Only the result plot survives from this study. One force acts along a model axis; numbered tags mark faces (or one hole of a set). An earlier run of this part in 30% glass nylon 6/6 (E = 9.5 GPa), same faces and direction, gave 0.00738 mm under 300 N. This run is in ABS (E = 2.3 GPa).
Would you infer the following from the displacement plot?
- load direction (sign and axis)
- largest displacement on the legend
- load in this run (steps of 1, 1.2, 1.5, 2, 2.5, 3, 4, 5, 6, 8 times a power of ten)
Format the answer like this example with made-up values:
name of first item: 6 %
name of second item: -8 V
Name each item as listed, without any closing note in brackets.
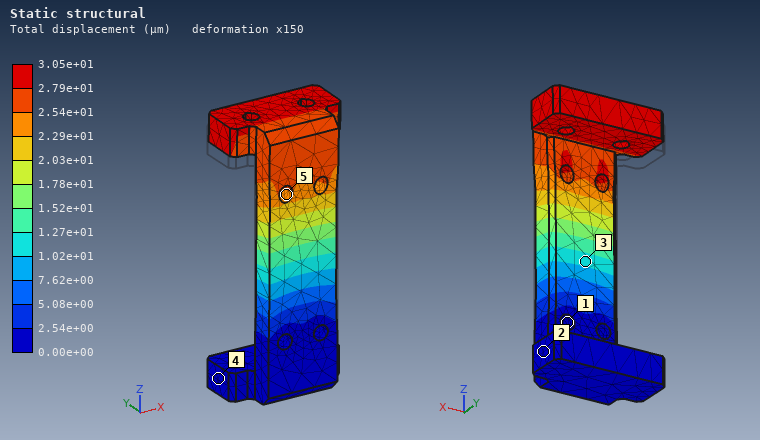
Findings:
load direction: +Z
largest displacement on the legend: 3.05e+01 µm
load in this run: 300 N
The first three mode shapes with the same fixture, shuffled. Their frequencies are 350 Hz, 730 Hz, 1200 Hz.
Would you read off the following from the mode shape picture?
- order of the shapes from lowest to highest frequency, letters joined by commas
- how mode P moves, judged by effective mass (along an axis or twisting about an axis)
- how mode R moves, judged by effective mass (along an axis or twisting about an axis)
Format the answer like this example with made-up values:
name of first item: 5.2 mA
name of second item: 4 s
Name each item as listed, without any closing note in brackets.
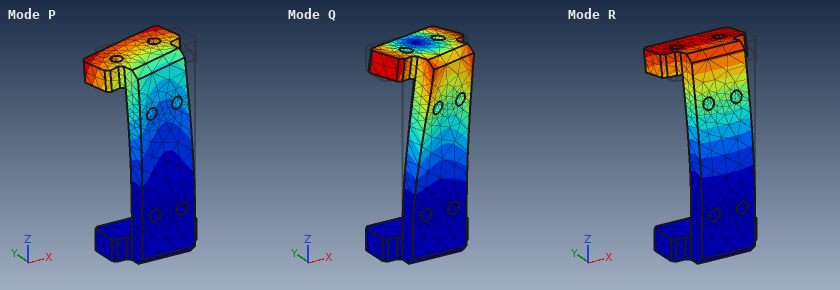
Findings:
order of the shapes from lowest to highest frequency, letters joined by commas: R, P, Q
how mode P moves, judged by effective mass: along X
how mode R moves, judged by effective mass: along Y
